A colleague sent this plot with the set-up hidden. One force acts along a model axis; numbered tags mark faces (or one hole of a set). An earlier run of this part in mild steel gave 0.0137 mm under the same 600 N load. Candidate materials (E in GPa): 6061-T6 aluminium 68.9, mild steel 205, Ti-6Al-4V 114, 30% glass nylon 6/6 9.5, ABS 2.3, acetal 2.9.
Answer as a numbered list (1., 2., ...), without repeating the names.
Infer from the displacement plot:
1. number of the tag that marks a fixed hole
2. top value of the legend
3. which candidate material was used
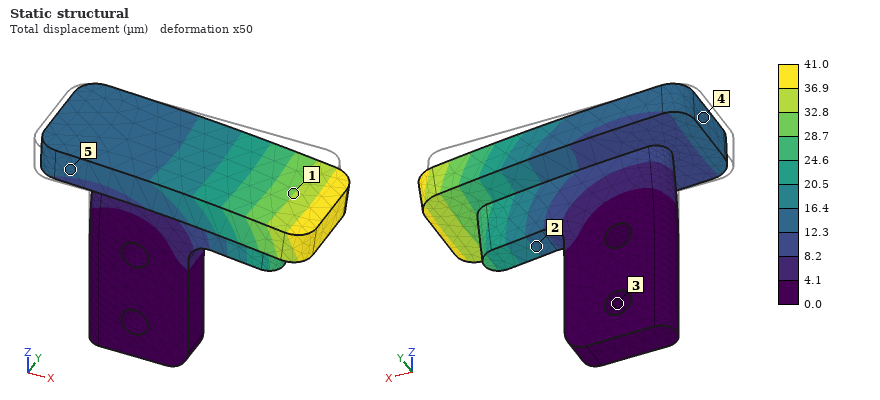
1. 3
2. 41.0 µm
3. 6061-T6 aluminium
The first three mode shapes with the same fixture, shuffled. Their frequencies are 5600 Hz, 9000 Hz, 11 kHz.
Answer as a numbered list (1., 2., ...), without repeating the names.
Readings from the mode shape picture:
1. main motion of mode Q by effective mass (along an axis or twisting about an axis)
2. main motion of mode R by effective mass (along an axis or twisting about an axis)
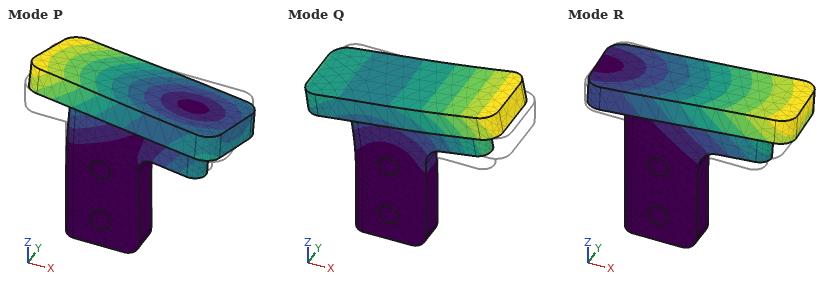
1. along X
2. along Y
